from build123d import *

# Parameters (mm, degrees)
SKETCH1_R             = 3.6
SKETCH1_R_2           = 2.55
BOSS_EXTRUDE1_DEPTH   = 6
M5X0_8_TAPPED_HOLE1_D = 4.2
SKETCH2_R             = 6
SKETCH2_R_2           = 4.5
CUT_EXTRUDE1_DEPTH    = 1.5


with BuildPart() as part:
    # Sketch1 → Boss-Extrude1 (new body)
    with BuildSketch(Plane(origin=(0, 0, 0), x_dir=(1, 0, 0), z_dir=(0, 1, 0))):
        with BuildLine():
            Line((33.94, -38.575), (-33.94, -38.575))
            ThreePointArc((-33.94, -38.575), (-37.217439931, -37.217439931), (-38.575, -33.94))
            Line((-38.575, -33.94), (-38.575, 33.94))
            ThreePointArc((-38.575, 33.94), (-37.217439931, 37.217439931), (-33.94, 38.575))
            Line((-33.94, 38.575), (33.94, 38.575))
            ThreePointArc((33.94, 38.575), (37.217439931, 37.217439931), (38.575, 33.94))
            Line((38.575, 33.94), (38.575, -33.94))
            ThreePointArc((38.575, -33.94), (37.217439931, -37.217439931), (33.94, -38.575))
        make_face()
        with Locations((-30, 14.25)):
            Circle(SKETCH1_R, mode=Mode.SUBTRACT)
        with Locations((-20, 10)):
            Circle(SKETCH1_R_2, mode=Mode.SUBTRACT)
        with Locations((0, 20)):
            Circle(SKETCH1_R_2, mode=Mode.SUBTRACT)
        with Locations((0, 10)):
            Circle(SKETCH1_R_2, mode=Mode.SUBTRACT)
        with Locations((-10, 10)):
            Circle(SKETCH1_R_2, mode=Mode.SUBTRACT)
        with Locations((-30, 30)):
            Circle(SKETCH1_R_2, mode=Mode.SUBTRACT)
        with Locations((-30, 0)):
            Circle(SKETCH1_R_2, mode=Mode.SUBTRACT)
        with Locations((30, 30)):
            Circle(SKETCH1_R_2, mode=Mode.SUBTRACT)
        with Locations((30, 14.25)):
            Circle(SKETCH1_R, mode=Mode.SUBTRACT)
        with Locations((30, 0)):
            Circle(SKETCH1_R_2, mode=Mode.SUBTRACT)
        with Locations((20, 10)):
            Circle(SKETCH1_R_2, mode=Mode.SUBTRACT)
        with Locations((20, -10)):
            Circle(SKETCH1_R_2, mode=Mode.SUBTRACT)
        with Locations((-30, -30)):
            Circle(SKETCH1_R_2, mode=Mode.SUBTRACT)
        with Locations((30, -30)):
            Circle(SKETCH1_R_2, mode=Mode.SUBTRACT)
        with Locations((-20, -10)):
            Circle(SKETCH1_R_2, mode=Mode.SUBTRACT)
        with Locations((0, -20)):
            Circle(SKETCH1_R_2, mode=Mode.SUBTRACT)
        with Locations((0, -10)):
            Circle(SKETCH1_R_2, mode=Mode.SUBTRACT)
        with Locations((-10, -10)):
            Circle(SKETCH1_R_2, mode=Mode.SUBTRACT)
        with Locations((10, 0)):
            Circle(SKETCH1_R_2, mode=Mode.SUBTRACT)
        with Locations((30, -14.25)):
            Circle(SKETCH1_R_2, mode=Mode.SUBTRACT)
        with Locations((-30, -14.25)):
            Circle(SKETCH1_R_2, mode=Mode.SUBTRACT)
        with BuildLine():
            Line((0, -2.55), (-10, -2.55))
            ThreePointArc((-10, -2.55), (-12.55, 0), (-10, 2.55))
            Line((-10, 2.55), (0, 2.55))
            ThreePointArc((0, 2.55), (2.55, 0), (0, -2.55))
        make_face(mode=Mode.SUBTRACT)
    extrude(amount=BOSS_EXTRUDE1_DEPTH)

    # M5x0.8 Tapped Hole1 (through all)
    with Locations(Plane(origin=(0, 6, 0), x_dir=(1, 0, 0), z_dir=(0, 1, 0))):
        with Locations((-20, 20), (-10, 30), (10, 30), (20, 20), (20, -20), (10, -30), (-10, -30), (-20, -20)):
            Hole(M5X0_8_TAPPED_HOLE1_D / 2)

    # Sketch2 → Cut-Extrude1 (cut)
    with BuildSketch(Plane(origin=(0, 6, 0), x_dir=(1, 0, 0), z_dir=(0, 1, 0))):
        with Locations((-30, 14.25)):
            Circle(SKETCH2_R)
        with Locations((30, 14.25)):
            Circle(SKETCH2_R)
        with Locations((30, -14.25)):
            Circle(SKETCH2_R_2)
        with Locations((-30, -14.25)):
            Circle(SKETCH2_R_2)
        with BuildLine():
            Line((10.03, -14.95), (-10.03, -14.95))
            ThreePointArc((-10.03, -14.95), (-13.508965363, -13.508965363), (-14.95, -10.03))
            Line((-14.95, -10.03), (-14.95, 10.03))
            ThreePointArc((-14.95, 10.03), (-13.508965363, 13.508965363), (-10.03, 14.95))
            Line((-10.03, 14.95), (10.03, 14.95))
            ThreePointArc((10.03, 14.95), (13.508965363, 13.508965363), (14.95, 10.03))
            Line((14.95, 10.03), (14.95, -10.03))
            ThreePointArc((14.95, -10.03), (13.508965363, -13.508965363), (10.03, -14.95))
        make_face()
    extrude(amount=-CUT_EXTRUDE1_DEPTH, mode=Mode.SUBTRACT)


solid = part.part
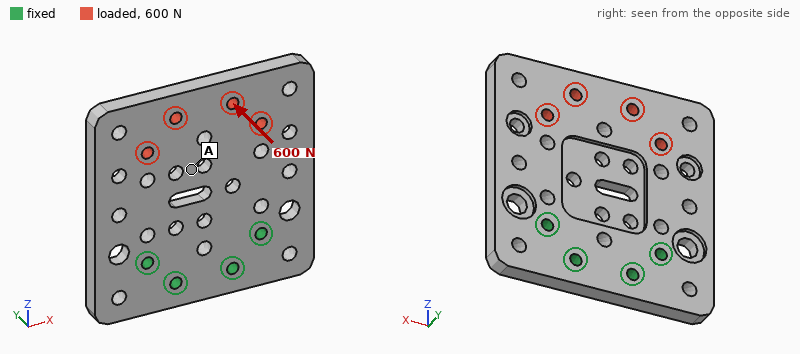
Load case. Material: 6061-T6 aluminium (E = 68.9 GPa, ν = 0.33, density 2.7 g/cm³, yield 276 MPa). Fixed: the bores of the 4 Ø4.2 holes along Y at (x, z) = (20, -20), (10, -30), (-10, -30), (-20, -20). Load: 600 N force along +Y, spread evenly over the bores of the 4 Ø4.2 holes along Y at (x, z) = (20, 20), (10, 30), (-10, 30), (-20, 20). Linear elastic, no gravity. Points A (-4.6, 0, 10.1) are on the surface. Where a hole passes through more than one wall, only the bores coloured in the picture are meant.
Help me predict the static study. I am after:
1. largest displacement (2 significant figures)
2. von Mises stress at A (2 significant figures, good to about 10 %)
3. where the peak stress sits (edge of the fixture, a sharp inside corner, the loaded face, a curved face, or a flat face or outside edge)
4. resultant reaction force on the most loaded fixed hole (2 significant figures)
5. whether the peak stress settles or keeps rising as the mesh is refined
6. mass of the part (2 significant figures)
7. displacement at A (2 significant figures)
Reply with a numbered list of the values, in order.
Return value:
1. 0.55 mm
2. 19 MPa
3. a sharp inside corner
4. 590 N
5. keeps rising
6. 82 g
7. 0.20 mm
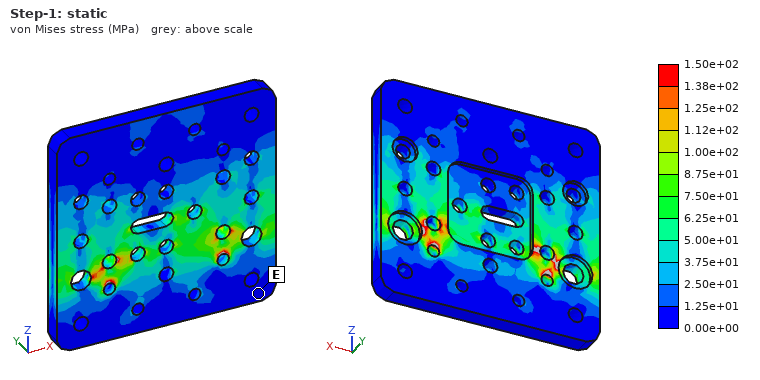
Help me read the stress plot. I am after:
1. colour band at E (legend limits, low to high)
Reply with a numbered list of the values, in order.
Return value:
1. 0.00e+00 to 1.25e+01 MPa
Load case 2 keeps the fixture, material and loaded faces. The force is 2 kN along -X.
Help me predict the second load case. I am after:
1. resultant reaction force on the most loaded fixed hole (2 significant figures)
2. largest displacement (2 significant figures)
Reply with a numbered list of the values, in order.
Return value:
1. 2.4 kN
2. 44 µm
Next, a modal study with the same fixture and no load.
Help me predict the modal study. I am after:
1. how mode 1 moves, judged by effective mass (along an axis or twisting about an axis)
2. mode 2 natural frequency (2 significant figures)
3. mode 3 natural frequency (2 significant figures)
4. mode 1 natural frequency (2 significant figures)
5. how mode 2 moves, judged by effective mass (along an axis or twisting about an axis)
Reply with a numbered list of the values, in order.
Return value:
1. along Y
2. 2200 Hz
3. 5600 Hz
4. 1100 Hz
5. twisting about Z
